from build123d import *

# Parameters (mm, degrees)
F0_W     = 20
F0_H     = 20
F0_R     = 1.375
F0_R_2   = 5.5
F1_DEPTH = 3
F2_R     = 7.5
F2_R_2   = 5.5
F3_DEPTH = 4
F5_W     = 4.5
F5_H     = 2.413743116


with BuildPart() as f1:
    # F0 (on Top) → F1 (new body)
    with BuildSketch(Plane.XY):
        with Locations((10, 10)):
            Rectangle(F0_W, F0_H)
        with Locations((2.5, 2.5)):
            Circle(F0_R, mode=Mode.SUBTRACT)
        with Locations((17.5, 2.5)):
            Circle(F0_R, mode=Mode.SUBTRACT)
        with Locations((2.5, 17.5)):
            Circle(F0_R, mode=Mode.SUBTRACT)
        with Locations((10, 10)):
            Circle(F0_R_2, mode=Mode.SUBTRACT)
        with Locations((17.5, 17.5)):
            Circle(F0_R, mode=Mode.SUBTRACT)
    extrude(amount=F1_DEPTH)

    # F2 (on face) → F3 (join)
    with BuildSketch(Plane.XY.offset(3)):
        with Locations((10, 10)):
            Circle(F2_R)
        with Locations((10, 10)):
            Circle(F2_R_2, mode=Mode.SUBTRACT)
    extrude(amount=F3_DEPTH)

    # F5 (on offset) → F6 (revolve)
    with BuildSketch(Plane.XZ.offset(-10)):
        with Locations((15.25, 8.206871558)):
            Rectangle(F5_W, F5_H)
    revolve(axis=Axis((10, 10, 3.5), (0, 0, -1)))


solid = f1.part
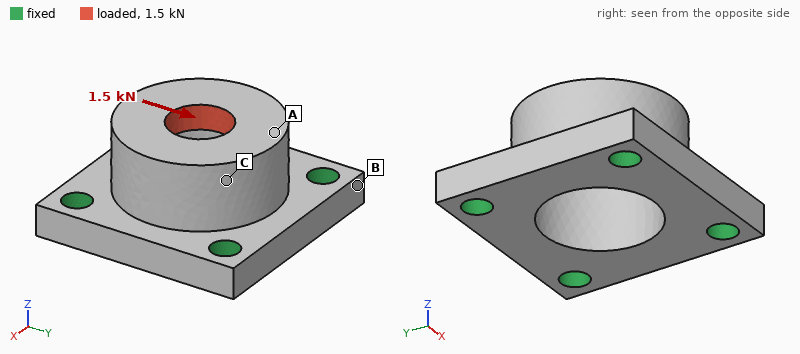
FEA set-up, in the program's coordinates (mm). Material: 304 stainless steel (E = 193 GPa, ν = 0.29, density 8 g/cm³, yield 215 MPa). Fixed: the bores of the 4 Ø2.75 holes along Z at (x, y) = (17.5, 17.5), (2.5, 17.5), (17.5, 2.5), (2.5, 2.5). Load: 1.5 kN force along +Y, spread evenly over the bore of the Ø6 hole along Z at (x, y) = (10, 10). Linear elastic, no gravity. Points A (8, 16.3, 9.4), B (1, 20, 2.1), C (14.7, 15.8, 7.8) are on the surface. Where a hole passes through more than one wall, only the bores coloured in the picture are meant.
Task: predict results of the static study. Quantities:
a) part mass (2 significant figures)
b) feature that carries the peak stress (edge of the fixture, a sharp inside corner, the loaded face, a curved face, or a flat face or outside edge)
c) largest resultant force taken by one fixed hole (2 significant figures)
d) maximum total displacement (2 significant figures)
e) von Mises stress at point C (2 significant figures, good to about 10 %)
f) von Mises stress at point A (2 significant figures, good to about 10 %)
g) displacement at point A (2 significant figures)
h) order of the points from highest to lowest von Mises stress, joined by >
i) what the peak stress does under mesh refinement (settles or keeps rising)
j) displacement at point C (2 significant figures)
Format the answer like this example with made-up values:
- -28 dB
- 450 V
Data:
- 12 g
- edge of the fixture
- 530 N
- 6.5 µm
- 21 MPa
- 41 MPa
- 6.2 µm
- A > C > B
- keeps rising
- 4.8 µm
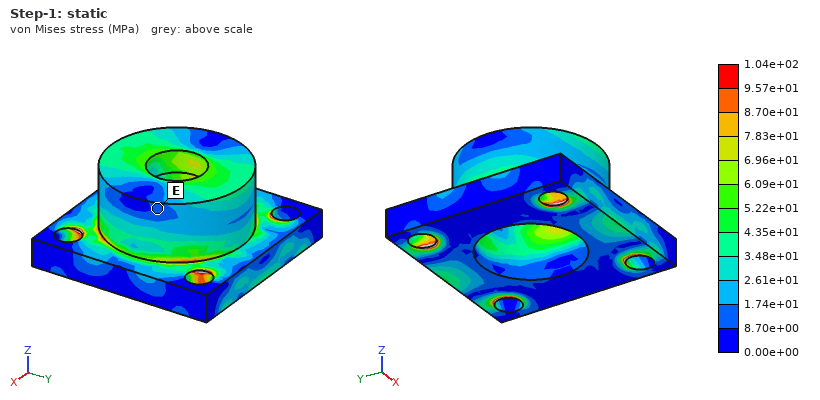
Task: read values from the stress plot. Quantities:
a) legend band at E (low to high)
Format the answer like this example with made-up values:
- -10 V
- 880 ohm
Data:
- 8.70e+00 to 1.74e+01 MPa
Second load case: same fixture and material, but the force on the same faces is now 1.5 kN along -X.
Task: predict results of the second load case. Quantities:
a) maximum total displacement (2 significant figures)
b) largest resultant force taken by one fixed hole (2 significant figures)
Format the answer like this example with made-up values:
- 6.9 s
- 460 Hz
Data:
- 6.5 µm
- 530 N
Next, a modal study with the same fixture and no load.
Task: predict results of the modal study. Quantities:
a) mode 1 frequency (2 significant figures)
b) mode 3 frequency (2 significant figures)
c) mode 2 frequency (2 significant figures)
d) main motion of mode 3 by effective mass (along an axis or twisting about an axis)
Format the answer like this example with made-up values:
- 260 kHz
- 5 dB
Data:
- 42 kHz
- 49 kHz
- 42 kHz
- along Z
